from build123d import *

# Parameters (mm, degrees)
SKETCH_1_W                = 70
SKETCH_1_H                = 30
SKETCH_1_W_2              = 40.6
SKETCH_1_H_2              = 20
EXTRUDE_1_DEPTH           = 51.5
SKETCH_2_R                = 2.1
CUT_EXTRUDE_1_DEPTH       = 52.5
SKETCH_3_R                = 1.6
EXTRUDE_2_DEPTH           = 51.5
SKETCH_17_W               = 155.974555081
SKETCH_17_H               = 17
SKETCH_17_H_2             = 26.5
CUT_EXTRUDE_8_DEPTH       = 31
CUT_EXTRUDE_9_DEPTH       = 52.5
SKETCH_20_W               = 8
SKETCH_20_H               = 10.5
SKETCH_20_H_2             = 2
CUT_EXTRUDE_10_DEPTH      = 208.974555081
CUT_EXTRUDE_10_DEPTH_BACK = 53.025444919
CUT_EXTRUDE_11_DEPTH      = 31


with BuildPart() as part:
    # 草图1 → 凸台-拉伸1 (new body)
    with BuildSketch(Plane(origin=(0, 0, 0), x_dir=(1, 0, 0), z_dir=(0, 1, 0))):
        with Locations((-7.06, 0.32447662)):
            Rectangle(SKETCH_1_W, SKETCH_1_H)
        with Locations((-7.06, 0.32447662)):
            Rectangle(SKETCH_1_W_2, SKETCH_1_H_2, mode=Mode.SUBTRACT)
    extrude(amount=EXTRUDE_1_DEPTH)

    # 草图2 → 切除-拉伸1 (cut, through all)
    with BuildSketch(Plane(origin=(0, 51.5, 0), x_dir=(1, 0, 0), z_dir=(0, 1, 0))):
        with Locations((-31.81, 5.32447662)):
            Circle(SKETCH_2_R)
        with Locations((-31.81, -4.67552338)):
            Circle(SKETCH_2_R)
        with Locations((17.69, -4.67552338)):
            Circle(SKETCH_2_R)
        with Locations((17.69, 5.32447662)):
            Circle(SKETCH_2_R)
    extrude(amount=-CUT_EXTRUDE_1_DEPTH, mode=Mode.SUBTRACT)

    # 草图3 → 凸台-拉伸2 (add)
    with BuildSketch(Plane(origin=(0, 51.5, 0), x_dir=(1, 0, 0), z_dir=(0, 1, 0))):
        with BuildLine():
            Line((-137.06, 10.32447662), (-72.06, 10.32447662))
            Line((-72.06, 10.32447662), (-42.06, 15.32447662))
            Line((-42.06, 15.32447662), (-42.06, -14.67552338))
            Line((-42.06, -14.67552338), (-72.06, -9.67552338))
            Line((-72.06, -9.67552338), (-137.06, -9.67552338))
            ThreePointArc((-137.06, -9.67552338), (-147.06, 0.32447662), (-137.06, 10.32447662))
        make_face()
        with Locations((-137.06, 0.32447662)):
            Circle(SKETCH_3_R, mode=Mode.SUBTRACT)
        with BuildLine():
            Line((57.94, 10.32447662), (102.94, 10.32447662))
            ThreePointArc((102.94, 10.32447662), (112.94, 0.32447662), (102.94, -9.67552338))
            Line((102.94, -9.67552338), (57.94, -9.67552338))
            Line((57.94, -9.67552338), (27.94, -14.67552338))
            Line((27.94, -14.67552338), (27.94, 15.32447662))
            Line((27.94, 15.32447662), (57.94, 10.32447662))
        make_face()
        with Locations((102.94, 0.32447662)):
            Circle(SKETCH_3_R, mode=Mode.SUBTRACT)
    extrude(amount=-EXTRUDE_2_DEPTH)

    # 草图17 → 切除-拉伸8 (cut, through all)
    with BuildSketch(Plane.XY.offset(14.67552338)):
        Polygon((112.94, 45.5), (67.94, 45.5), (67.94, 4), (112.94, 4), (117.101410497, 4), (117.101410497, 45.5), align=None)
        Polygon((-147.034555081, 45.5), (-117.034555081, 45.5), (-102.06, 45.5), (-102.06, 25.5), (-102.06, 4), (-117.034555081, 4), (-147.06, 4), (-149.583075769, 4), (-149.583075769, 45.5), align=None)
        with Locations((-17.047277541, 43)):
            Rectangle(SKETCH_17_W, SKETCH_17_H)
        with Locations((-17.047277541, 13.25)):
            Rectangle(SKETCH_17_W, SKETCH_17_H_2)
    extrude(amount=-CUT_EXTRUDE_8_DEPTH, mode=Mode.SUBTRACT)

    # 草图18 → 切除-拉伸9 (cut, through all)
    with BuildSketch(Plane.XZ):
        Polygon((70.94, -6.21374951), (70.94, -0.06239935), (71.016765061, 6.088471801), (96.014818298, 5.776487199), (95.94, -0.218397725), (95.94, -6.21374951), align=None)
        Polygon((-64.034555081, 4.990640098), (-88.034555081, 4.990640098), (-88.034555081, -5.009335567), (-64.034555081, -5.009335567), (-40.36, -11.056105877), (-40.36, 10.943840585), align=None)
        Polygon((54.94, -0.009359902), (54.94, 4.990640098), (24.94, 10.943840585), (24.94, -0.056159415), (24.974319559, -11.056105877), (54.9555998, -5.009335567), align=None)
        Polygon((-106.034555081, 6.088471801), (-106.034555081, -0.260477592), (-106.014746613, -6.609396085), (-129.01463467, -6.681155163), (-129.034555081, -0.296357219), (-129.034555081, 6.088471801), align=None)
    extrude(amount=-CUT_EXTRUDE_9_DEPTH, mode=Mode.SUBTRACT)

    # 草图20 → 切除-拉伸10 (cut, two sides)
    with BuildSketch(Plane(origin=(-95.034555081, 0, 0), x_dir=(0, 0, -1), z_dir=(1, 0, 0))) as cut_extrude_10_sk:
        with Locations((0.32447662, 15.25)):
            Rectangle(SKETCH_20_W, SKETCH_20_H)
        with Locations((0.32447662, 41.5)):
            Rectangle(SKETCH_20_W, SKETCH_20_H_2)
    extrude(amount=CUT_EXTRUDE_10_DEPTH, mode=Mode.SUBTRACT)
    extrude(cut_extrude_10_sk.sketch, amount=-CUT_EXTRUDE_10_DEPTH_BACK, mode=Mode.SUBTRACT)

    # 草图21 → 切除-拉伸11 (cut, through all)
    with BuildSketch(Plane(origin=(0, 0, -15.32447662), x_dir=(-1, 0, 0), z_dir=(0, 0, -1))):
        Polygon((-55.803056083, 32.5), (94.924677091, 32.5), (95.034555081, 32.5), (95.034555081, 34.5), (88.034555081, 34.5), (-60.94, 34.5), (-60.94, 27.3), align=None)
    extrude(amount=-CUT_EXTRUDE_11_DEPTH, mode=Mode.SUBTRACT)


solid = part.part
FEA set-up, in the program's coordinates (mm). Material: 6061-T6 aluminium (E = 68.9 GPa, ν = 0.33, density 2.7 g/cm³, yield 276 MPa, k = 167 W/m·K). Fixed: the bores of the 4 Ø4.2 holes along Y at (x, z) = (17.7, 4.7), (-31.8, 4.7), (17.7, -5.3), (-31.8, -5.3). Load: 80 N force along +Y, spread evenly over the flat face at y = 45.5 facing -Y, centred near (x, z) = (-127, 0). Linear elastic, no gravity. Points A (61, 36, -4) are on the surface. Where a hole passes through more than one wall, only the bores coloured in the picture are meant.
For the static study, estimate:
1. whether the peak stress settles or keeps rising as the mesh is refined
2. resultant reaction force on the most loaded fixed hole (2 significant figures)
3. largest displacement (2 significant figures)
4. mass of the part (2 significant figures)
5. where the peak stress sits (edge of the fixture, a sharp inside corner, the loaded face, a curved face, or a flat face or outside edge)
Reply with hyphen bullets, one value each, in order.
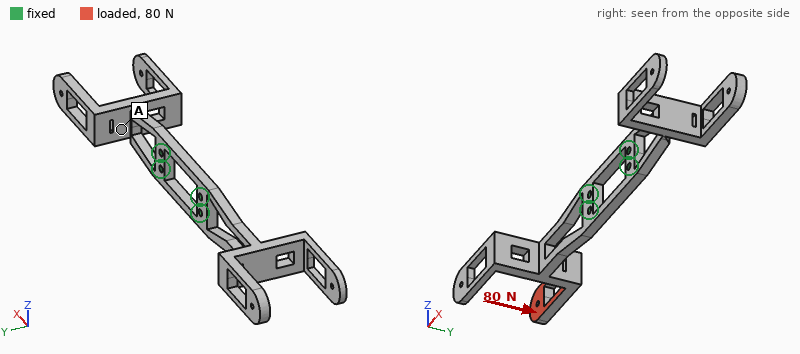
- keeps rising
- 51 N
- 2.4 mm
- 99 g
- a sharp inside corner
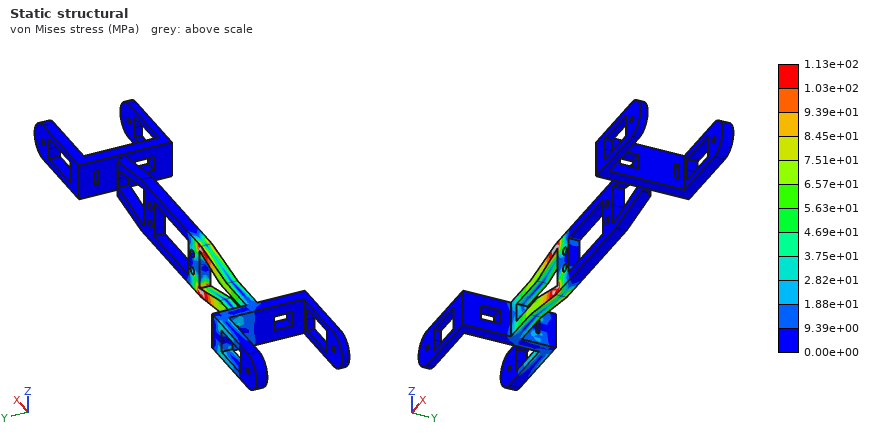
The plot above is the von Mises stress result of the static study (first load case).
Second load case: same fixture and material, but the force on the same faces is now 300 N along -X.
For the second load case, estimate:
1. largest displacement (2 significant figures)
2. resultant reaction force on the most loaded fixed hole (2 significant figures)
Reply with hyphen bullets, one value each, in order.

- 2.0 mm
- 140 N
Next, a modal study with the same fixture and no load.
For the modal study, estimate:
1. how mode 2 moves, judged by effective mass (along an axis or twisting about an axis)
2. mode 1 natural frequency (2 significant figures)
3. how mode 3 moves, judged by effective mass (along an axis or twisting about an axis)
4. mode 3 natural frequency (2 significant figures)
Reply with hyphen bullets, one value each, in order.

- along Y
- 220 Hz
- twisting about X
- 570 Hz
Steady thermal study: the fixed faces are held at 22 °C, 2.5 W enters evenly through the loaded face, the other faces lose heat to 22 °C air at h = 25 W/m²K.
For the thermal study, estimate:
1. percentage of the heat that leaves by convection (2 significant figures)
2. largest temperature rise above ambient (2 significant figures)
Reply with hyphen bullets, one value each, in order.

- 59 %
- 14 K
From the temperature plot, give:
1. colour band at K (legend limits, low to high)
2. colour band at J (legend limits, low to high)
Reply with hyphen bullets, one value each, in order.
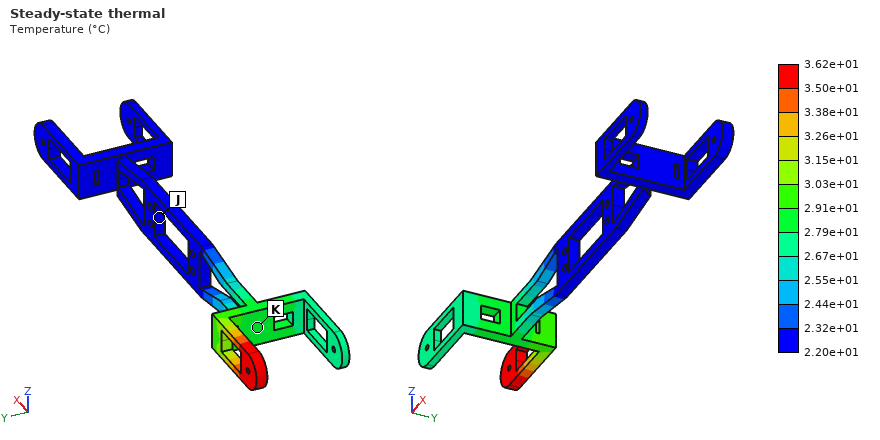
- 2.79e+01 to 2.91e+01 °C
- 2.20e+01 to 2.32e+01 °C
